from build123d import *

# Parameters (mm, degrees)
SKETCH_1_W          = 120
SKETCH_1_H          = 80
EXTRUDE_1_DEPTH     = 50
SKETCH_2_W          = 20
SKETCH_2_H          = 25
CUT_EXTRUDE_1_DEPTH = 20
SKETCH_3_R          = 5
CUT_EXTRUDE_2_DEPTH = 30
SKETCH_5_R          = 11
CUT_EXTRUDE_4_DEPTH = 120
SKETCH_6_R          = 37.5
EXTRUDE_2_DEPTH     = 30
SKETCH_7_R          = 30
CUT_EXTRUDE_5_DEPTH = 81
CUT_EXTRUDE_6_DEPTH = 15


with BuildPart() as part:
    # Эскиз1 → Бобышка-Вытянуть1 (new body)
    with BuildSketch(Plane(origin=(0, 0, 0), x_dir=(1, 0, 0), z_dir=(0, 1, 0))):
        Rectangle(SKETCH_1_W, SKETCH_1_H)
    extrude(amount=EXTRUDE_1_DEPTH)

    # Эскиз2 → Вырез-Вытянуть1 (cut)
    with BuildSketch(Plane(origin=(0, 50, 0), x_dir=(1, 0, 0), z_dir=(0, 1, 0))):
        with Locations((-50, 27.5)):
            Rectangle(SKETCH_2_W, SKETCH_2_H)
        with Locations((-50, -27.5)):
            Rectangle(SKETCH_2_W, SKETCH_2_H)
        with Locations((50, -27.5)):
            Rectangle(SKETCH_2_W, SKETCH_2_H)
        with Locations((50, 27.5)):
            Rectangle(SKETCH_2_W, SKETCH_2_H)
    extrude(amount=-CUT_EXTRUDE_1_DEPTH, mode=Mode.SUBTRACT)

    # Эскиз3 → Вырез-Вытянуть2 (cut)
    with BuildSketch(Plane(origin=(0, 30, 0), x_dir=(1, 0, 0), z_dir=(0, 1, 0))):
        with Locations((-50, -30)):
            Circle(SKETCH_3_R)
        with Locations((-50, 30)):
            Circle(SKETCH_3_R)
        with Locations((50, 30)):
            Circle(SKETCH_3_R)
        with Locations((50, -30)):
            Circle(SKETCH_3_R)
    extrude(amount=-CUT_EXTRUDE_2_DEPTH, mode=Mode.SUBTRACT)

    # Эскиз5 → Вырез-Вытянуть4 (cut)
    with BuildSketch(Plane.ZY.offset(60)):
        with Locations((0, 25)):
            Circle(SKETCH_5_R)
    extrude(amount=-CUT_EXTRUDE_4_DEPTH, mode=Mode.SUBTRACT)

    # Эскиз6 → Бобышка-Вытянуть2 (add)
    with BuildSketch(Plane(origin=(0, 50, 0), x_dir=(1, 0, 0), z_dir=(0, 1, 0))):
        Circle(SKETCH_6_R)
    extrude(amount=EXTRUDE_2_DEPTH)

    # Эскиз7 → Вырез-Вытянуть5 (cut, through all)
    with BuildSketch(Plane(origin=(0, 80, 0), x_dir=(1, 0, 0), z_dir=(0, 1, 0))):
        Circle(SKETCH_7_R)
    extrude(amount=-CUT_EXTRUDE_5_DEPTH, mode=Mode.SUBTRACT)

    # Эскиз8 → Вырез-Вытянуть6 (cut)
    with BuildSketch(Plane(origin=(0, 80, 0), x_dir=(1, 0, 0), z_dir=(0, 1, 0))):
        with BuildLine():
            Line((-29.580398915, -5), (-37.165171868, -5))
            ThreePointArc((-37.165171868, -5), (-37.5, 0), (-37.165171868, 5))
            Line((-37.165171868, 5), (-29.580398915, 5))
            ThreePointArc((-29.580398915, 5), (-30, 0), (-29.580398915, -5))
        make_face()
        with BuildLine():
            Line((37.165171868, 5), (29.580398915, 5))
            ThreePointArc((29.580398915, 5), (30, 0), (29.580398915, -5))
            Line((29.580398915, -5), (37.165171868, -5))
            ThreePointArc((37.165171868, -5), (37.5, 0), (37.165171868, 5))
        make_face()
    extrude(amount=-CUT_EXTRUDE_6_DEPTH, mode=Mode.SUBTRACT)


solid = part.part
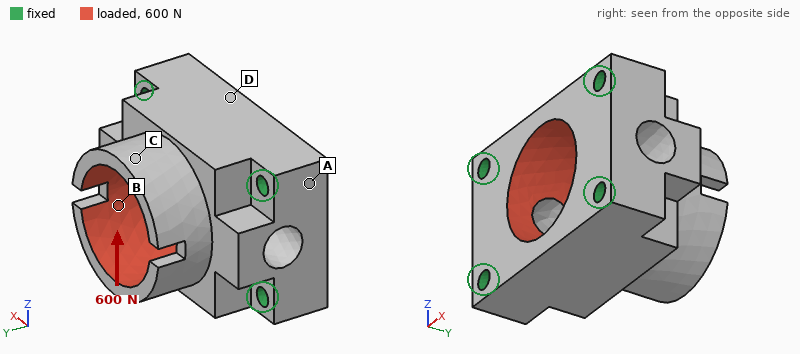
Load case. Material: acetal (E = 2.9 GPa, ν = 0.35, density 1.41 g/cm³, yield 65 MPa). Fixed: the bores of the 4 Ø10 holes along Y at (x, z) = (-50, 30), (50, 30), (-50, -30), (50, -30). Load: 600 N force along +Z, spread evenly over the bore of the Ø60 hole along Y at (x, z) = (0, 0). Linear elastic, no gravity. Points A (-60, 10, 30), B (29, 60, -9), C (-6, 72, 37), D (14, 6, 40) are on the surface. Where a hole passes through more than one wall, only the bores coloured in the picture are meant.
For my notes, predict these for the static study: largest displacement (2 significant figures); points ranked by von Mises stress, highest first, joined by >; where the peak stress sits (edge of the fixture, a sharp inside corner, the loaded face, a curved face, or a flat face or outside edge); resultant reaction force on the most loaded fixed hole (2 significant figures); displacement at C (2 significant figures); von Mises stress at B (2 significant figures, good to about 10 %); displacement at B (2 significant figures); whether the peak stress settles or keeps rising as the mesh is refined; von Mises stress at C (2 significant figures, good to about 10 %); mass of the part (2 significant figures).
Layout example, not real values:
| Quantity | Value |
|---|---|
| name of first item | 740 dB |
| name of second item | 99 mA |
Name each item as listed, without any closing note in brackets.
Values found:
| Quantity | Value |
|---|---|
| largest displacement | 25 µm |
| points ranked by von Mises stress, highest first, joined by > | B > C > D > A |
| where the peak stress sits | edge of the fixture |
| resultant reaction force on the most loaded fixed hole | 190 N |
| displacement at C | 22 µm |
| von Mises stress at B | 0.51 MPa |
| displacement at B | 12 µm |
| whether the peak stress settles or keeps rising as the mesh is refined | keeps rising |
| von Mises stress at C | 0.29 MPa |
| mass of the part | 440 g |
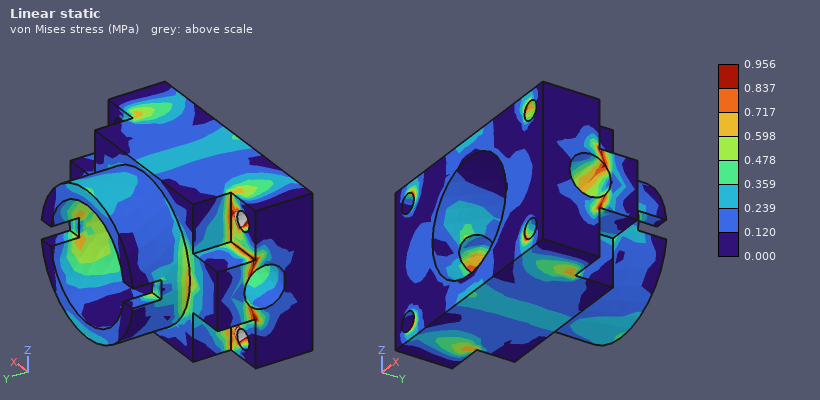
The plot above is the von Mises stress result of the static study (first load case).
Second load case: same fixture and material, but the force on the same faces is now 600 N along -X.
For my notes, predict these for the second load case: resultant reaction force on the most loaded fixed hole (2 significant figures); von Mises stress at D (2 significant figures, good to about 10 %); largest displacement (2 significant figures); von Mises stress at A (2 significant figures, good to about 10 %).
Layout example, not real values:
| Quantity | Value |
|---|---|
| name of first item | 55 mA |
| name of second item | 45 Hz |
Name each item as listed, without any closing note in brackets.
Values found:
| Quantity | Value |
|---|---|
| resultant reaction force on the most loaded fixed hole | 170 N |
| von Mises stress at D | 0.10 MPa |
| largest displacement | 20 µm |
| von Mises stress at A | 0.10 MPa |
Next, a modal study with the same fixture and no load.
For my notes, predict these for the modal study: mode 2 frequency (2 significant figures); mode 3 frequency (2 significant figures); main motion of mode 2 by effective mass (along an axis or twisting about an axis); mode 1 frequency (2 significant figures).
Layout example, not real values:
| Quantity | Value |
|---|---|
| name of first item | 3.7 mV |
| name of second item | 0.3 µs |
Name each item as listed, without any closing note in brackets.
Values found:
| Quantity | Value |
|---|---|
| mode 2 frequency | 2100 Hz |
| mode 3 frequency | 2500 Hz |
| main motion of mode 2 by effective mass | along Z |
| mode 1 frequency | 2000 Hz |
